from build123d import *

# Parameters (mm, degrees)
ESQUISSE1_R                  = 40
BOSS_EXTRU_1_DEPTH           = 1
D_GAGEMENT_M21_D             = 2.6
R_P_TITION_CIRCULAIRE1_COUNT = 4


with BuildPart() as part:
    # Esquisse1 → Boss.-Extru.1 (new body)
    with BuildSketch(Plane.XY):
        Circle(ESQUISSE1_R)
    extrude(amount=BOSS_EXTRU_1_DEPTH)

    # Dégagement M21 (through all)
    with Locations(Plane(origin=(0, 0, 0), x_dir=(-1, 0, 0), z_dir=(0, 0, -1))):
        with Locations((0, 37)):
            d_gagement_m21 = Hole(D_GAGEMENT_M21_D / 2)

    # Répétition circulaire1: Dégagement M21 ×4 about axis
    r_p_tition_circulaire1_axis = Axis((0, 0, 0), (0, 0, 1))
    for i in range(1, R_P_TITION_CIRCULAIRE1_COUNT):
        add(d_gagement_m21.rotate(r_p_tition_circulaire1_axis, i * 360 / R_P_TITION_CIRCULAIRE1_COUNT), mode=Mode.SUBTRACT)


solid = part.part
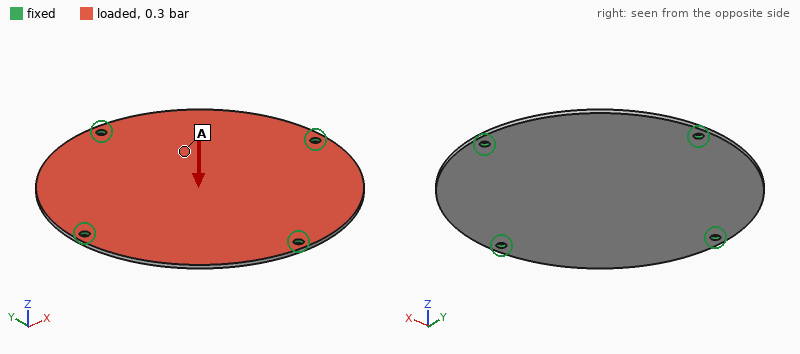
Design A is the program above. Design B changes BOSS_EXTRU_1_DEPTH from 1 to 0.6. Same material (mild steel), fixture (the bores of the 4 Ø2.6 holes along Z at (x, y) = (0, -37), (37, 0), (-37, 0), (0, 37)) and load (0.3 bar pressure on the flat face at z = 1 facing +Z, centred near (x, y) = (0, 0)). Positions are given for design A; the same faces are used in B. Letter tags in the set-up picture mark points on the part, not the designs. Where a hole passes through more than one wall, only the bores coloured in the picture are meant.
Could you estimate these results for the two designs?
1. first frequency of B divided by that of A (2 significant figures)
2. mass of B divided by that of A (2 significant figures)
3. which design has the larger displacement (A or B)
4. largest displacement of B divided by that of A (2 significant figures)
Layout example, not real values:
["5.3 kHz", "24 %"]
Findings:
["0.61", "0.60", "B", "4.5"]
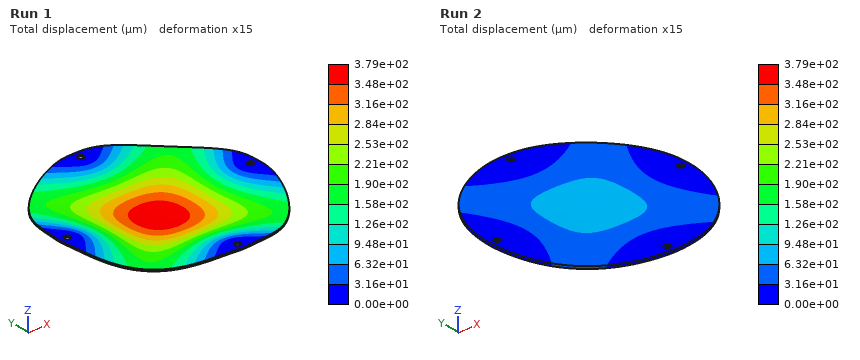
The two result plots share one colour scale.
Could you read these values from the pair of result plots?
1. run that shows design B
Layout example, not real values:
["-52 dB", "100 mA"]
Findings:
["Run 1"]
